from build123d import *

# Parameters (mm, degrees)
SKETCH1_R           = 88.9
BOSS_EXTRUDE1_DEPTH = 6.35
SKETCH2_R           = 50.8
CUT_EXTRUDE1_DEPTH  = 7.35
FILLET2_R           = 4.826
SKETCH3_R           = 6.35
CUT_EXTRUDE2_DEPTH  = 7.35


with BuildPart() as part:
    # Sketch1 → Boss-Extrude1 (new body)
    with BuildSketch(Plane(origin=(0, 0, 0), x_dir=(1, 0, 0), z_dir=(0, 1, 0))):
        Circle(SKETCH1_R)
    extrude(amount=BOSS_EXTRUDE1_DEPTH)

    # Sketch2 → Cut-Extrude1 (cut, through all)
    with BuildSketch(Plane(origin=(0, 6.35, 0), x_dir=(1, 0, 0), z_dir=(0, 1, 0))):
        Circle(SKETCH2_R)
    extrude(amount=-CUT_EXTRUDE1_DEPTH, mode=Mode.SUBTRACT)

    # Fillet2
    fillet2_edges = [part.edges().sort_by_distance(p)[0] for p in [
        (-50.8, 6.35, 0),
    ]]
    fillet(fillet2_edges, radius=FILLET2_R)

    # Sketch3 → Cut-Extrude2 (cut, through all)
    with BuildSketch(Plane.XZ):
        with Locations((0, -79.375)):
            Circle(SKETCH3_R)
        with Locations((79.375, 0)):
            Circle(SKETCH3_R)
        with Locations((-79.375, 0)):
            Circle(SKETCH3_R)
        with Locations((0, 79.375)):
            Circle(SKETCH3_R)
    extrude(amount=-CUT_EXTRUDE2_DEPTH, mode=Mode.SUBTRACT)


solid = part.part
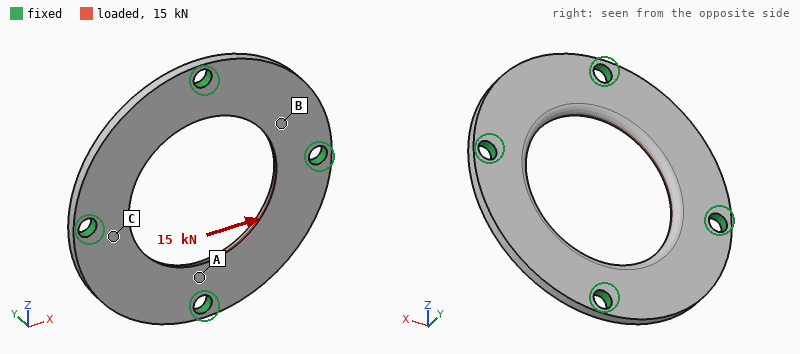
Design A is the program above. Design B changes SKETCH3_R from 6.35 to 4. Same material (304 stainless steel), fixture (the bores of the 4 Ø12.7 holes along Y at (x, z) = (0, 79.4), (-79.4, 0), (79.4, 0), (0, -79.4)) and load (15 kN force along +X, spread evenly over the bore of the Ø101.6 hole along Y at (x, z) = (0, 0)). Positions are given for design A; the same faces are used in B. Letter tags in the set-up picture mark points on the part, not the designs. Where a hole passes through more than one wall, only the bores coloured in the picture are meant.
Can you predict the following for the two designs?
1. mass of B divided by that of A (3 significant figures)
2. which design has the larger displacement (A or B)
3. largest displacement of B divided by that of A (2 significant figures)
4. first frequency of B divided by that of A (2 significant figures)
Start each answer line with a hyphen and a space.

- 1.02
- B
- 1.2
- 0.87
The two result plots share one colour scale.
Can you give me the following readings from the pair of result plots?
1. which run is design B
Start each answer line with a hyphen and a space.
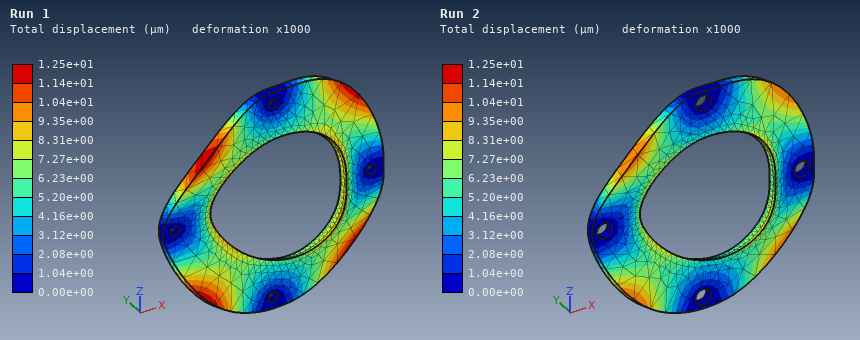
- Run 1
